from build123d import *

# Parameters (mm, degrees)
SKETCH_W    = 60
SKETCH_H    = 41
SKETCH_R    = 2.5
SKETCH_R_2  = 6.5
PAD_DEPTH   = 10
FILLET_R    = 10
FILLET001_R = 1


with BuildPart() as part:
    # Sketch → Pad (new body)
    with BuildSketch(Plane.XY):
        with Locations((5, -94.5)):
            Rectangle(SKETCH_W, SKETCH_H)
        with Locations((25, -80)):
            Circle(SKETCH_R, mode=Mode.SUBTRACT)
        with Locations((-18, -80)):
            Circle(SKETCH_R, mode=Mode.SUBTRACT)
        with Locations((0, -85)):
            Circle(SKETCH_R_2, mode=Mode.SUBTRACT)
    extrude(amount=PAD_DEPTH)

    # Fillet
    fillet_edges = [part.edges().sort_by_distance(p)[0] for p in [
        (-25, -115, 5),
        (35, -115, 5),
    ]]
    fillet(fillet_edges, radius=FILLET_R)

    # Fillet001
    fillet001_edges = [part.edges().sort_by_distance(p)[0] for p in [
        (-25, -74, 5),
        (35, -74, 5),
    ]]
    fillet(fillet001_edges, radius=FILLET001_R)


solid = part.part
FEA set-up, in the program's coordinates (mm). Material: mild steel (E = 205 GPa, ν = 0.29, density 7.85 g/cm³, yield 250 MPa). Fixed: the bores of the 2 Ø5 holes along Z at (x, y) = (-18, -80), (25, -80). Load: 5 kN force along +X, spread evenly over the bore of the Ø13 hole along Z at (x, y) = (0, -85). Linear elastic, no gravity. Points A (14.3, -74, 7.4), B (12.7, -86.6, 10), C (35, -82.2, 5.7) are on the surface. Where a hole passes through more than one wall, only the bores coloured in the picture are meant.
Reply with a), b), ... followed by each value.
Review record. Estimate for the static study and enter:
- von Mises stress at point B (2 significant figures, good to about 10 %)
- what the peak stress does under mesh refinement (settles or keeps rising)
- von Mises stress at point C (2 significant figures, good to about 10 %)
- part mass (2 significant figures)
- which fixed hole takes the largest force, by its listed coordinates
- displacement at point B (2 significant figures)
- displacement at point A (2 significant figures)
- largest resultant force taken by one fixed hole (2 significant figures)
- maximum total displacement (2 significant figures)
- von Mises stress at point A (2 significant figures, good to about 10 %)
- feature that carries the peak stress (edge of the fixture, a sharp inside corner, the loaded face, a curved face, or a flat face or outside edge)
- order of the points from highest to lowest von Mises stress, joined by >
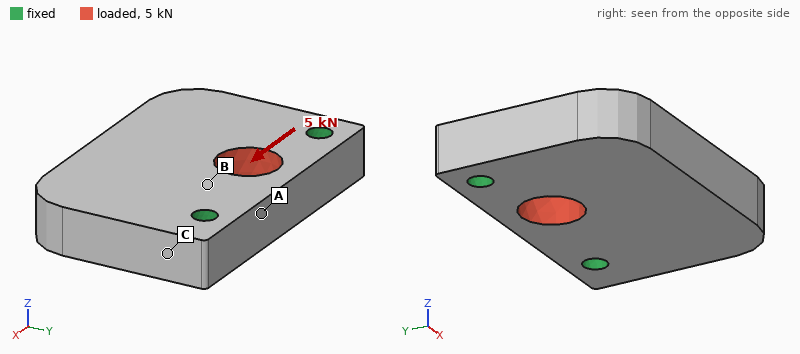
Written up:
a) 14 MPa
b) keeps rising
c) 4.1 MPa
d) 180 g
e) (-18, -80)
f) 1.2 µm
g) 0.56 µm
h) 2.7 kN
i) 2.1 µm
j) 10 MPa
k) edge of the fixture
l) B > A > C
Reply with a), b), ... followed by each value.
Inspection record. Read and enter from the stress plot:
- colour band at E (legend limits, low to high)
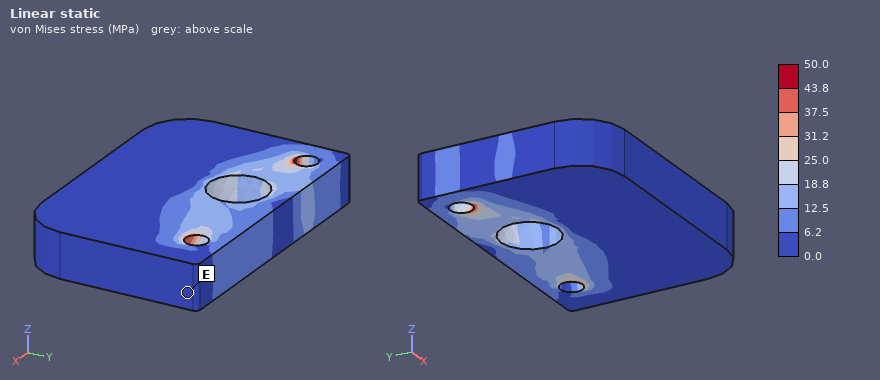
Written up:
a) 0.0 to 6.2 MPa
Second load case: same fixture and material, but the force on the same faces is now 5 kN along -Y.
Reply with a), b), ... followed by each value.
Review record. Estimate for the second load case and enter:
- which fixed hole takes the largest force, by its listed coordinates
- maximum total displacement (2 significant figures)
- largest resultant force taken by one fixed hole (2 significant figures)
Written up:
a) (-18, -80)
b) 4.4 µm
c) 3.0 kN
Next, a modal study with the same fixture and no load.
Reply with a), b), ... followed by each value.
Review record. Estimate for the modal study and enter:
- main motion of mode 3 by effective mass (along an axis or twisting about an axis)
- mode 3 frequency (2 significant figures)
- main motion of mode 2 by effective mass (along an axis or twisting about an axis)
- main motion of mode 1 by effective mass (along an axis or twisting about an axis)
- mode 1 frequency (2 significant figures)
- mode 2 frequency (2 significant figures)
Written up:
a) along X
b) 16 kHz
c) twisting about Y
d) along Z
e) 5300 Hz
f) 10 kHz
